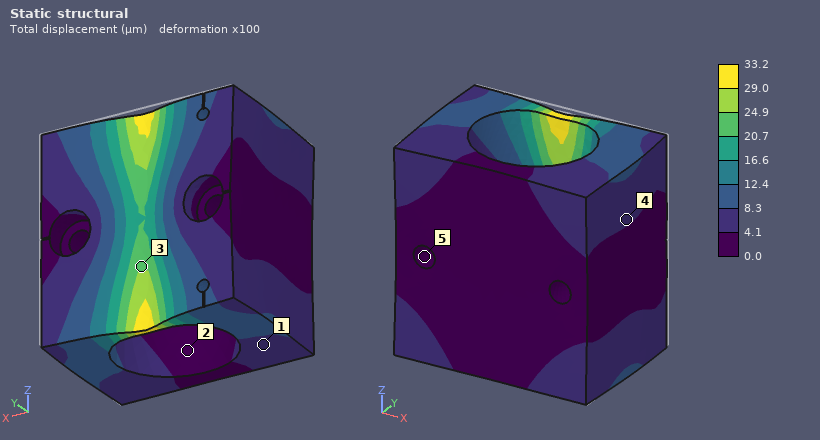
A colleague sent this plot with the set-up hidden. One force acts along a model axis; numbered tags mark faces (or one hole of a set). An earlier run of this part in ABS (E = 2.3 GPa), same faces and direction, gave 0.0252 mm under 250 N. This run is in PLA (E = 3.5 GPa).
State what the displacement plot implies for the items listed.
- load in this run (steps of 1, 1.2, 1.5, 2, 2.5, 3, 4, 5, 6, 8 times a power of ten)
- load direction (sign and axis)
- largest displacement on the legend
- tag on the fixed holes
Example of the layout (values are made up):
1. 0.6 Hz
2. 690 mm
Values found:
1. 500 N
2. -Y
3. 33.2 µm
4. 5
